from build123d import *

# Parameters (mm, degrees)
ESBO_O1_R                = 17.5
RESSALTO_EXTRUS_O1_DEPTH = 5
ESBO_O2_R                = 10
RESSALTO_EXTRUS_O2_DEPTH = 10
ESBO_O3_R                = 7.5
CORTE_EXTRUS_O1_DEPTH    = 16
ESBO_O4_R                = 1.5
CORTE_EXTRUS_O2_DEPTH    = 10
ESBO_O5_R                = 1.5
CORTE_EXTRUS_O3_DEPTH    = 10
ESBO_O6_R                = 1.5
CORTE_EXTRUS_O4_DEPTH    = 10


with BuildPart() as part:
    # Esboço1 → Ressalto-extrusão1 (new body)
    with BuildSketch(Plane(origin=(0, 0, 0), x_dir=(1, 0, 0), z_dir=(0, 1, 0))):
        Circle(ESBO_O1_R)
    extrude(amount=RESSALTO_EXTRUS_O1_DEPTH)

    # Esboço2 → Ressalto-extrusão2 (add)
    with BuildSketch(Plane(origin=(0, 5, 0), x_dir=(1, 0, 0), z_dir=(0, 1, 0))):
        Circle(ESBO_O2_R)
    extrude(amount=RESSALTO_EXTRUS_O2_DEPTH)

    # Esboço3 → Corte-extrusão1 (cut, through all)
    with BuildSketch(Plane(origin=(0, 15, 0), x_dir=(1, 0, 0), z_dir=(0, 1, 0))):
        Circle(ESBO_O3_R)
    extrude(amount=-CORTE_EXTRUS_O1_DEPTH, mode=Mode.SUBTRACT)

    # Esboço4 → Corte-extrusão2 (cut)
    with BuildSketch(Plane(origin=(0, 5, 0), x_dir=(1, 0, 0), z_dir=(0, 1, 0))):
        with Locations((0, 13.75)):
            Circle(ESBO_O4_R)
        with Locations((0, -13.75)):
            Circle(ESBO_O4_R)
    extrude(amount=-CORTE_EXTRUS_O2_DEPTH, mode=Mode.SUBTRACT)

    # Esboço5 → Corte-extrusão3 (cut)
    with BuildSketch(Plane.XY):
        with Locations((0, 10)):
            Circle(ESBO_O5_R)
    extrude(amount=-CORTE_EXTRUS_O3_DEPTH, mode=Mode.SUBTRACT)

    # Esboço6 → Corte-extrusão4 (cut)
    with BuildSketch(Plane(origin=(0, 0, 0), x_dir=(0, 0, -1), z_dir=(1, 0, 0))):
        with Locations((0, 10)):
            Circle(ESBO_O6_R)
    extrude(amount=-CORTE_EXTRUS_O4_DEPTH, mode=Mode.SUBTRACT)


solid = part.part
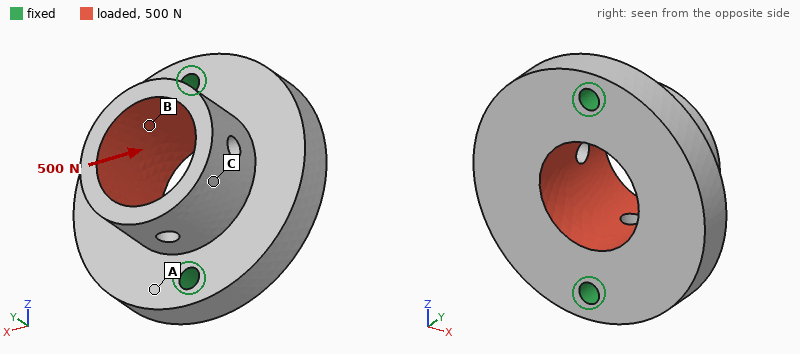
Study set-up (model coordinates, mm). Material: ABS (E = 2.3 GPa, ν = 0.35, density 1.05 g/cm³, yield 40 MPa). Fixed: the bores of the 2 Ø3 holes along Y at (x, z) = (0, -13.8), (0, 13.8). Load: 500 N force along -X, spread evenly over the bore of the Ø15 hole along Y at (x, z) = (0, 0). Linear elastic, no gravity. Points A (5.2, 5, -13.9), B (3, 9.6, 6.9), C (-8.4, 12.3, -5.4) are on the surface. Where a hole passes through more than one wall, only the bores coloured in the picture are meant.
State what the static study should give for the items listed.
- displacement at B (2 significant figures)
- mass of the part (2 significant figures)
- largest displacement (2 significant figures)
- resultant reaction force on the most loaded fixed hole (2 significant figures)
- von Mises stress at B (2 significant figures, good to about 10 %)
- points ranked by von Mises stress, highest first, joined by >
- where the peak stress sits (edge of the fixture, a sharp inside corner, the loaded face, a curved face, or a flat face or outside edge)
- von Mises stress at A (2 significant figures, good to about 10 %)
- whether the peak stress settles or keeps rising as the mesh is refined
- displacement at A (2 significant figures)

0.15 mm
5.5 g
0.31 mm
250 N
6.5 MPa
A > B > C
edge of the fixture
11 MPa
keeps rising
0.050 mm
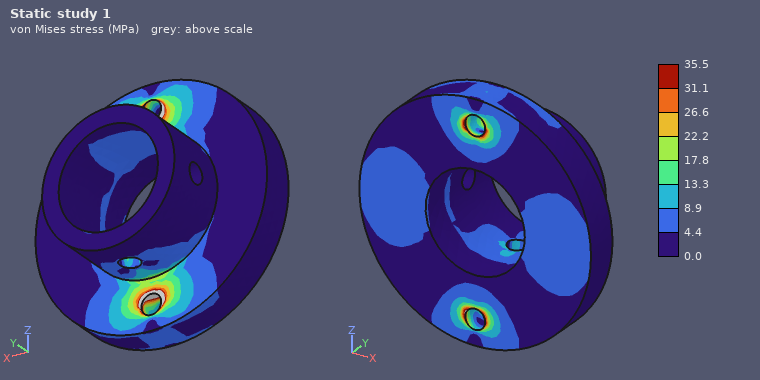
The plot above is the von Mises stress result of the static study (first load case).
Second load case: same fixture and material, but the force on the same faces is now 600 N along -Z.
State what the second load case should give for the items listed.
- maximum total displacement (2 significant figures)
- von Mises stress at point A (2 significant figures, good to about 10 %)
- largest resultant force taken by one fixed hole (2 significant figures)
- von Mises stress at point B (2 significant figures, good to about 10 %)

99 µm
3.0 MPa
320 N
5.1 MPa
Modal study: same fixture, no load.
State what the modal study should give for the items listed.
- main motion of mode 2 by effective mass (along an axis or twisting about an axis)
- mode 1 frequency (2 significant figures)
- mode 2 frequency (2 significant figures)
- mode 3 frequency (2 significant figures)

along Y
2800 Hz
4400 Hz
7800 Hz
